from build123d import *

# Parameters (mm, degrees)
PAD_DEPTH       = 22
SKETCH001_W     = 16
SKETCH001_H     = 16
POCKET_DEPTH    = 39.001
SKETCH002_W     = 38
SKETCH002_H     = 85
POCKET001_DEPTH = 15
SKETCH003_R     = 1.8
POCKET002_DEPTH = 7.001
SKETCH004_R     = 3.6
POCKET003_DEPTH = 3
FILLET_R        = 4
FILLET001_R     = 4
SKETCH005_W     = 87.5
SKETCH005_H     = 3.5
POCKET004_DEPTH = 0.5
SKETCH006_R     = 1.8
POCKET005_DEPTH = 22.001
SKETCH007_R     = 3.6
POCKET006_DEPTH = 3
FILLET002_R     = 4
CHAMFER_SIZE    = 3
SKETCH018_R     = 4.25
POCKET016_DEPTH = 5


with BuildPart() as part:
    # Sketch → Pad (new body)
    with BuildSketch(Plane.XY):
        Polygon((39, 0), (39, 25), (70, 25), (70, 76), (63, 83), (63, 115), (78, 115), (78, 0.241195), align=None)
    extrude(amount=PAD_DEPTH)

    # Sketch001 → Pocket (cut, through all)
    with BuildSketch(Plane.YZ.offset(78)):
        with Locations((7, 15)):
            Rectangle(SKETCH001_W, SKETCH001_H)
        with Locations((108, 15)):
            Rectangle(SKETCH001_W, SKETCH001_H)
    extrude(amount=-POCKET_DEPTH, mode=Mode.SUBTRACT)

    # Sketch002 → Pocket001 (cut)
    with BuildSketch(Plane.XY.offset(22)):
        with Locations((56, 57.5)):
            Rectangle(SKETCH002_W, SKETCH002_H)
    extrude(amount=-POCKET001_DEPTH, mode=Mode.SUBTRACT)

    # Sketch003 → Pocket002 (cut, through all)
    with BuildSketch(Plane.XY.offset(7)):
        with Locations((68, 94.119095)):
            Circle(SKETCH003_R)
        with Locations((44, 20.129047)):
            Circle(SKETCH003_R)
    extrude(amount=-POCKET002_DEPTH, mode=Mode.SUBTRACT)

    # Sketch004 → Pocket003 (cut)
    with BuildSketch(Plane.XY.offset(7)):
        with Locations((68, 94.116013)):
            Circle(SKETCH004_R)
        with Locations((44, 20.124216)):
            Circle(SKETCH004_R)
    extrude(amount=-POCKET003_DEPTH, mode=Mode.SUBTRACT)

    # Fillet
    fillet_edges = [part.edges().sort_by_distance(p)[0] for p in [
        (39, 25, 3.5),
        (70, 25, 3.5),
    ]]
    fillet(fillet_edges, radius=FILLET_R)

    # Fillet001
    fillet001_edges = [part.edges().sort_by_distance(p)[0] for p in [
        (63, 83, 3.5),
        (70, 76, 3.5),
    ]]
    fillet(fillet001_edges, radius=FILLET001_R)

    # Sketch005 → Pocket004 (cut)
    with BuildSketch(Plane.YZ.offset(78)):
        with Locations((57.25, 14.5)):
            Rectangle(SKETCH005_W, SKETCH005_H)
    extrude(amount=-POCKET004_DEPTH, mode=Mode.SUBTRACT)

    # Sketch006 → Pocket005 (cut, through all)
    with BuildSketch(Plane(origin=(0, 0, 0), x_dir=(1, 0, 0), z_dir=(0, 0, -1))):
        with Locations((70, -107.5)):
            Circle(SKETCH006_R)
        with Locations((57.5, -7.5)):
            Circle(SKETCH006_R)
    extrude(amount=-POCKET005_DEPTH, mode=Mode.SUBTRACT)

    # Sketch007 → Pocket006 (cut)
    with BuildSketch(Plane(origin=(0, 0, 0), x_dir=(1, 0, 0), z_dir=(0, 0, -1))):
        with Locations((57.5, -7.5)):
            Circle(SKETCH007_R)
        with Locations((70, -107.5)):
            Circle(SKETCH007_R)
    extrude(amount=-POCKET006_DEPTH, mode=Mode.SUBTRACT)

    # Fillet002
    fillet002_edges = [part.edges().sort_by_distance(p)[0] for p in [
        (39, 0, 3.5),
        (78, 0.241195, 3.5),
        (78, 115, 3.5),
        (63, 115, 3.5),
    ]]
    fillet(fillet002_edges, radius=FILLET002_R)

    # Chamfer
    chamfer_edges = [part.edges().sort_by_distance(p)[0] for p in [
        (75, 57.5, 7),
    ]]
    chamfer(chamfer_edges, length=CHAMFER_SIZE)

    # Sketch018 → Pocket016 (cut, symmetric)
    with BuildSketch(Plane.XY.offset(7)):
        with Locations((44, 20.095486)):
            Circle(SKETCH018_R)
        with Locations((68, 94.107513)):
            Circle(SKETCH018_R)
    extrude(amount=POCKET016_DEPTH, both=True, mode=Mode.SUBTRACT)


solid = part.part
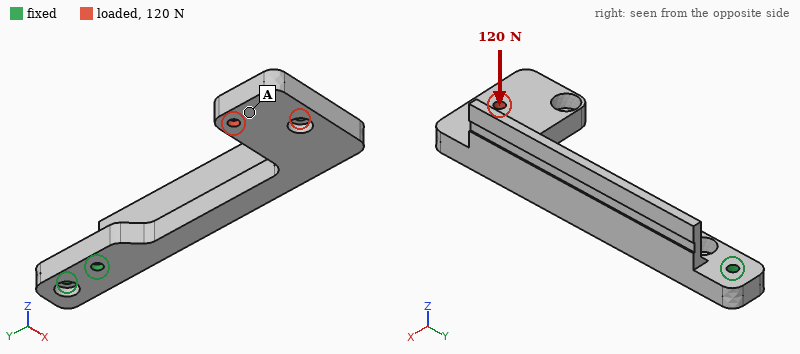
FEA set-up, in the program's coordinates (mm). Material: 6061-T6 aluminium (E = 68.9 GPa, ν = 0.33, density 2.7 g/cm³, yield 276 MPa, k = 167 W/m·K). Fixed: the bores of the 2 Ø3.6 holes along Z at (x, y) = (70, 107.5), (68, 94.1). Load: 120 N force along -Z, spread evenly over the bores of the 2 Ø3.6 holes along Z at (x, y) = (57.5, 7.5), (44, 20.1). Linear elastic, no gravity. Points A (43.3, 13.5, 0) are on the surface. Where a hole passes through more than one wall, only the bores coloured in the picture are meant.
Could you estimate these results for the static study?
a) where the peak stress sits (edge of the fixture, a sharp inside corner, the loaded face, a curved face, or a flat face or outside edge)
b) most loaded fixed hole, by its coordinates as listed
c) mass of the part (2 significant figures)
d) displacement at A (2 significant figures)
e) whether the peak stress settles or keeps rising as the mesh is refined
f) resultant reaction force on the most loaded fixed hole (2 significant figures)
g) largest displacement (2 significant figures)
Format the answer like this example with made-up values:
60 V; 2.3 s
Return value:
edge of the fixture; (68, 94.1); 45 g; 0.61 mm; keeps rising; 810 N; 0.70 mm
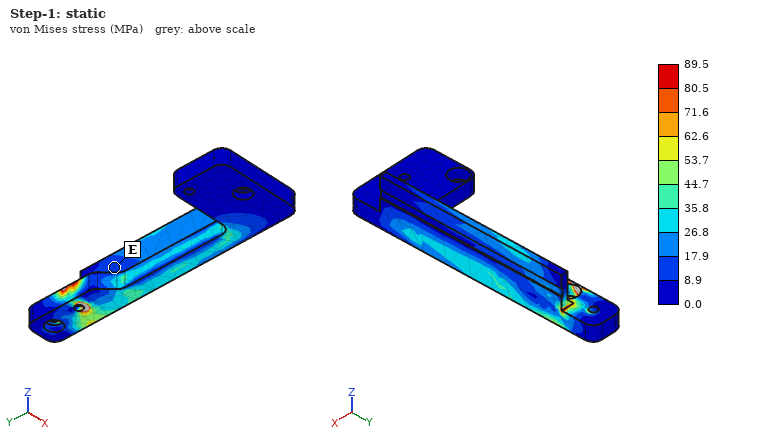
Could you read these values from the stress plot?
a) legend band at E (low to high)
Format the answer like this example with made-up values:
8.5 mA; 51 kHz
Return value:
8.9 to 17.9 MPa
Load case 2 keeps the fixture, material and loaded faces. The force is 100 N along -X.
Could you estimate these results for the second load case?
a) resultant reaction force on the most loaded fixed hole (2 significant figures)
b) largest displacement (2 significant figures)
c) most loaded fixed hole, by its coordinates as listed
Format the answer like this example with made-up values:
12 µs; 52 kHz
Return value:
550 N; 0.76 mm; (68, 94.1)
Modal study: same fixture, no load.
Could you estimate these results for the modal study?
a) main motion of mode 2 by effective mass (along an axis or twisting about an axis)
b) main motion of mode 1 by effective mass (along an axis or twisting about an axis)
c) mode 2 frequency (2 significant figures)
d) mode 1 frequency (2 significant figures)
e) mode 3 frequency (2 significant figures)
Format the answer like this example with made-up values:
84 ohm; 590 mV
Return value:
along Z; along X; 660 Hz; 440 Hz; 1300 Hz
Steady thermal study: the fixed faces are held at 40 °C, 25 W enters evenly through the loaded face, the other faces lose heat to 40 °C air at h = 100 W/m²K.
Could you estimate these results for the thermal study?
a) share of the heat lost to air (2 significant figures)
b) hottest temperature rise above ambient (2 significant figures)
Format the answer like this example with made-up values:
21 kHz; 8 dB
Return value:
79 %; 55 K
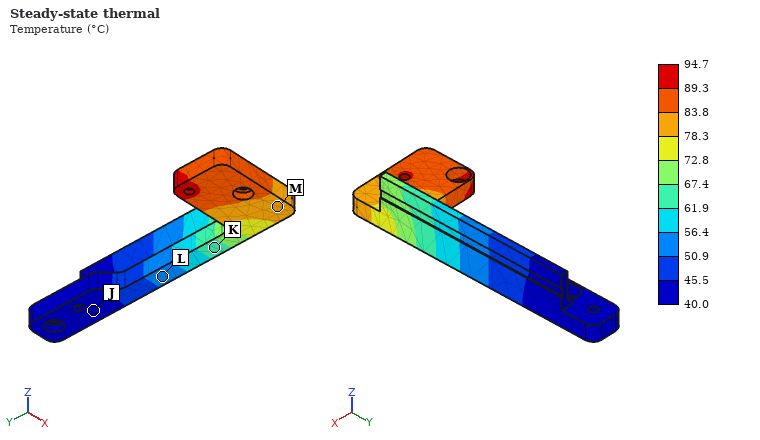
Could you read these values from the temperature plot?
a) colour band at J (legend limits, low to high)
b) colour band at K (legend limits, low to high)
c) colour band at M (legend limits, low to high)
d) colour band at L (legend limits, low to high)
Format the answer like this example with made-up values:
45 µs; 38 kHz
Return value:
40.0 to 45.5 °C; 61.9 to 67.4 °C; 78.3 to 83.8 °C; 50.9 to 56.4 °C
